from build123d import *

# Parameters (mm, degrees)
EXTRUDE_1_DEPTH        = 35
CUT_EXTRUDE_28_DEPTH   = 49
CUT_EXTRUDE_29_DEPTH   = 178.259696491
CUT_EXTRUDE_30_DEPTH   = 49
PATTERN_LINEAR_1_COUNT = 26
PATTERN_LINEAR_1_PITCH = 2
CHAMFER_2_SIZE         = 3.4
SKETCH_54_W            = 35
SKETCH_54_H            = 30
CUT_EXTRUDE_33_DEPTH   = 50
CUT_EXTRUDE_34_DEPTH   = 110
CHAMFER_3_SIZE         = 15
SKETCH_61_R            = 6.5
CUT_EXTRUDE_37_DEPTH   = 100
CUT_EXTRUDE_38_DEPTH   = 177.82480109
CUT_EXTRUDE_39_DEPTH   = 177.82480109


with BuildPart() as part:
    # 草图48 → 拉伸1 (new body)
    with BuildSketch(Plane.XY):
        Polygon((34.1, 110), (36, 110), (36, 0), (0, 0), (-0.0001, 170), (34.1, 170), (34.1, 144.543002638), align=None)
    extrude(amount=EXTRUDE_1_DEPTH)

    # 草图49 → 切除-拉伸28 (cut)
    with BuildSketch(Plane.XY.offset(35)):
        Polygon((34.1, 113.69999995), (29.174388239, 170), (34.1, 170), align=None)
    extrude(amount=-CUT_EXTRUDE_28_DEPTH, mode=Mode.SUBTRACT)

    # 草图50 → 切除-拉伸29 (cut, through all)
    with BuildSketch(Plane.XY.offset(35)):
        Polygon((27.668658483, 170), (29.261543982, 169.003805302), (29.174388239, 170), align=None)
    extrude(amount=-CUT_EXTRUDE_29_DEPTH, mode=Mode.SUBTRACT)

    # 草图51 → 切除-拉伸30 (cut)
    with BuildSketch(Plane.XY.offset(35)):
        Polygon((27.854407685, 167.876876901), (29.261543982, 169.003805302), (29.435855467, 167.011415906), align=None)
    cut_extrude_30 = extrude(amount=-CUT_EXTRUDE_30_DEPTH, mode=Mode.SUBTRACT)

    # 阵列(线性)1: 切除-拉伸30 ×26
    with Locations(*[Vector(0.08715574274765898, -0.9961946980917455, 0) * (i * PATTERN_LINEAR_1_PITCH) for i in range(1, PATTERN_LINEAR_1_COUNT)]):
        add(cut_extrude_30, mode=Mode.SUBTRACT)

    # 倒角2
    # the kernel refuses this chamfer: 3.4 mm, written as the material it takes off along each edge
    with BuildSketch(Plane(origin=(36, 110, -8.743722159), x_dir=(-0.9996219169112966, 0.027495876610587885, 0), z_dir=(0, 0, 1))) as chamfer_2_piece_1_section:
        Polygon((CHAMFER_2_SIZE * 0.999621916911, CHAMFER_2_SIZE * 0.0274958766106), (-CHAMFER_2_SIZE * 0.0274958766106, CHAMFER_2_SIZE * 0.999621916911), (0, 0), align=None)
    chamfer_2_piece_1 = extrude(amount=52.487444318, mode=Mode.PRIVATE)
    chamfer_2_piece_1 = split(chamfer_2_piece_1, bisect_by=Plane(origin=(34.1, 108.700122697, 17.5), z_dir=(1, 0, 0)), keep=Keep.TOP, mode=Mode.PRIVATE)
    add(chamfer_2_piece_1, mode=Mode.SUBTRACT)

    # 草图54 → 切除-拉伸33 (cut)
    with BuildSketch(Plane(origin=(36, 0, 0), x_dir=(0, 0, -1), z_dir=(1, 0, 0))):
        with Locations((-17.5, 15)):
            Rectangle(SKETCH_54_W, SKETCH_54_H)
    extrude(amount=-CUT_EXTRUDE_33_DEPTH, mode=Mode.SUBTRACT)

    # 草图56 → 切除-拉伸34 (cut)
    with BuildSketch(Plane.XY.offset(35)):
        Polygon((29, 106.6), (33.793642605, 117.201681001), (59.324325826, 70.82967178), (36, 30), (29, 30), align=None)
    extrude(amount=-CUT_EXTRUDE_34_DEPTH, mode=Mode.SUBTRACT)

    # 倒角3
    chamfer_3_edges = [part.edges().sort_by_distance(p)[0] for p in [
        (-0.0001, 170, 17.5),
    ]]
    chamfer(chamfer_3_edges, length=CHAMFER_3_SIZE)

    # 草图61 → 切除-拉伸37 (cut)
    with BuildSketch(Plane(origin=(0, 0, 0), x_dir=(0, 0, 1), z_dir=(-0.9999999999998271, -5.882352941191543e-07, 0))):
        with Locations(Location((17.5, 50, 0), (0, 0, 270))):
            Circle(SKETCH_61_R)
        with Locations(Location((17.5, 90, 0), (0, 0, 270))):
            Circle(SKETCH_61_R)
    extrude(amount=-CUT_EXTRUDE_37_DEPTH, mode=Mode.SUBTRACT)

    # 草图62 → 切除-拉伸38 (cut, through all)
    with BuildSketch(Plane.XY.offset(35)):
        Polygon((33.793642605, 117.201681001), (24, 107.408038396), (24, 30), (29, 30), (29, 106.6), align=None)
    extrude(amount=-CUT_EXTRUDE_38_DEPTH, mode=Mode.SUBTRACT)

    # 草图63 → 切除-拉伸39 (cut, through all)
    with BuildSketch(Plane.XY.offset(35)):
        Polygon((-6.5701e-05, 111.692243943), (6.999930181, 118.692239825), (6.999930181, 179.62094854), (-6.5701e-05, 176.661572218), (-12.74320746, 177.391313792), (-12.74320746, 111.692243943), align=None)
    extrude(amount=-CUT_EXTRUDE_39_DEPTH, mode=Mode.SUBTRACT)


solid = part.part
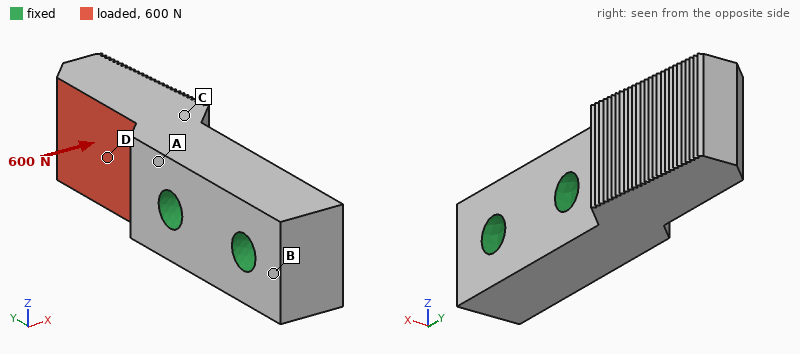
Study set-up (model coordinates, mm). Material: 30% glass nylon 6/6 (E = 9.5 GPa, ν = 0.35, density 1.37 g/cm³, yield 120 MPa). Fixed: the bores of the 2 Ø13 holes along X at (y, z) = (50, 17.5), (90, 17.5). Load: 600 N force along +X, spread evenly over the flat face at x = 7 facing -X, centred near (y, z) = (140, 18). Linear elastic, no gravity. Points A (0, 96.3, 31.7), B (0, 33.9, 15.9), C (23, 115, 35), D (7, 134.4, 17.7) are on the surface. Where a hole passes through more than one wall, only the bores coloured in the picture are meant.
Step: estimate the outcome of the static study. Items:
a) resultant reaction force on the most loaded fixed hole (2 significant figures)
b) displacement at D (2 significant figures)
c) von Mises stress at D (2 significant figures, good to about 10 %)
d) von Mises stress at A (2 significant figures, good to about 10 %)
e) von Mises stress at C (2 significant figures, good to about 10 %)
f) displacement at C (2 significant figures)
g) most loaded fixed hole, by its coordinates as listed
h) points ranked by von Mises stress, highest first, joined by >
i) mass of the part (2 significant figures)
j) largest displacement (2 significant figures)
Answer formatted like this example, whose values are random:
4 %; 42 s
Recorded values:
690 N; 0.063 mm; 1.7 MPa; 4.7 MPa; 3.3 MPa; 0.026 mm; (90, 17.5); A > C > D > B; 150 g; 0.14 mm
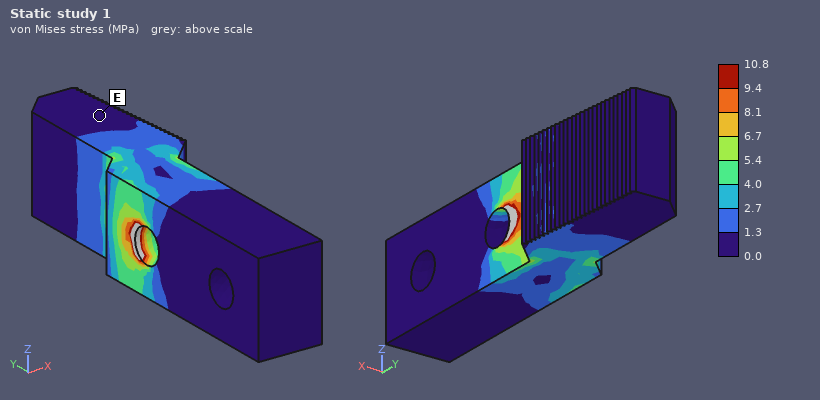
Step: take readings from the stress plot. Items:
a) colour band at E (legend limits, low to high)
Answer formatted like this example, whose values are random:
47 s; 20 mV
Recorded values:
0.0 to 1.3 MPa
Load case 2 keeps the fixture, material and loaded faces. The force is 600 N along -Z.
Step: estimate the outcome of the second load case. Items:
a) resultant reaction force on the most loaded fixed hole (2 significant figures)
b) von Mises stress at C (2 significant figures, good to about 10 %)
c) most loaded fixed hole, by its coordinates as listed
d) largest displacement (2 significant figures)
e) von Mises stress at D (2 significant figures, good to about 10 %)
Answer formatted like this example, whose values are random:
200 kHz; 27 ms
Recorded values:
880 N; 3.6 MPa; (90, 17.5); 0.11 mm; 3.2 MPa
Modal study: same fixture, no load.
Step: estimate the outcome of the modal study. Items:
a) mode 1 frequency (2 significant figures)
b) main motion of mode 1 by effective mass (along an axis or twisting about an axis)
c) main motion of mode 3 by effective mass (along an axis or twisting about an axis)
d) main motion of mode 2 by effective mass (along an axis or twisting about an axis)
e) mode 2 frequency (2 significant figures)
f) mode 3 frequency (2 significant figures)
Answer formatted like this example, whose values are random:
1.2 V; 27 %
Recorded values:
1600 Hz; along X; twisting about Y; along Z; 1900 Hz; 4500 Hz
